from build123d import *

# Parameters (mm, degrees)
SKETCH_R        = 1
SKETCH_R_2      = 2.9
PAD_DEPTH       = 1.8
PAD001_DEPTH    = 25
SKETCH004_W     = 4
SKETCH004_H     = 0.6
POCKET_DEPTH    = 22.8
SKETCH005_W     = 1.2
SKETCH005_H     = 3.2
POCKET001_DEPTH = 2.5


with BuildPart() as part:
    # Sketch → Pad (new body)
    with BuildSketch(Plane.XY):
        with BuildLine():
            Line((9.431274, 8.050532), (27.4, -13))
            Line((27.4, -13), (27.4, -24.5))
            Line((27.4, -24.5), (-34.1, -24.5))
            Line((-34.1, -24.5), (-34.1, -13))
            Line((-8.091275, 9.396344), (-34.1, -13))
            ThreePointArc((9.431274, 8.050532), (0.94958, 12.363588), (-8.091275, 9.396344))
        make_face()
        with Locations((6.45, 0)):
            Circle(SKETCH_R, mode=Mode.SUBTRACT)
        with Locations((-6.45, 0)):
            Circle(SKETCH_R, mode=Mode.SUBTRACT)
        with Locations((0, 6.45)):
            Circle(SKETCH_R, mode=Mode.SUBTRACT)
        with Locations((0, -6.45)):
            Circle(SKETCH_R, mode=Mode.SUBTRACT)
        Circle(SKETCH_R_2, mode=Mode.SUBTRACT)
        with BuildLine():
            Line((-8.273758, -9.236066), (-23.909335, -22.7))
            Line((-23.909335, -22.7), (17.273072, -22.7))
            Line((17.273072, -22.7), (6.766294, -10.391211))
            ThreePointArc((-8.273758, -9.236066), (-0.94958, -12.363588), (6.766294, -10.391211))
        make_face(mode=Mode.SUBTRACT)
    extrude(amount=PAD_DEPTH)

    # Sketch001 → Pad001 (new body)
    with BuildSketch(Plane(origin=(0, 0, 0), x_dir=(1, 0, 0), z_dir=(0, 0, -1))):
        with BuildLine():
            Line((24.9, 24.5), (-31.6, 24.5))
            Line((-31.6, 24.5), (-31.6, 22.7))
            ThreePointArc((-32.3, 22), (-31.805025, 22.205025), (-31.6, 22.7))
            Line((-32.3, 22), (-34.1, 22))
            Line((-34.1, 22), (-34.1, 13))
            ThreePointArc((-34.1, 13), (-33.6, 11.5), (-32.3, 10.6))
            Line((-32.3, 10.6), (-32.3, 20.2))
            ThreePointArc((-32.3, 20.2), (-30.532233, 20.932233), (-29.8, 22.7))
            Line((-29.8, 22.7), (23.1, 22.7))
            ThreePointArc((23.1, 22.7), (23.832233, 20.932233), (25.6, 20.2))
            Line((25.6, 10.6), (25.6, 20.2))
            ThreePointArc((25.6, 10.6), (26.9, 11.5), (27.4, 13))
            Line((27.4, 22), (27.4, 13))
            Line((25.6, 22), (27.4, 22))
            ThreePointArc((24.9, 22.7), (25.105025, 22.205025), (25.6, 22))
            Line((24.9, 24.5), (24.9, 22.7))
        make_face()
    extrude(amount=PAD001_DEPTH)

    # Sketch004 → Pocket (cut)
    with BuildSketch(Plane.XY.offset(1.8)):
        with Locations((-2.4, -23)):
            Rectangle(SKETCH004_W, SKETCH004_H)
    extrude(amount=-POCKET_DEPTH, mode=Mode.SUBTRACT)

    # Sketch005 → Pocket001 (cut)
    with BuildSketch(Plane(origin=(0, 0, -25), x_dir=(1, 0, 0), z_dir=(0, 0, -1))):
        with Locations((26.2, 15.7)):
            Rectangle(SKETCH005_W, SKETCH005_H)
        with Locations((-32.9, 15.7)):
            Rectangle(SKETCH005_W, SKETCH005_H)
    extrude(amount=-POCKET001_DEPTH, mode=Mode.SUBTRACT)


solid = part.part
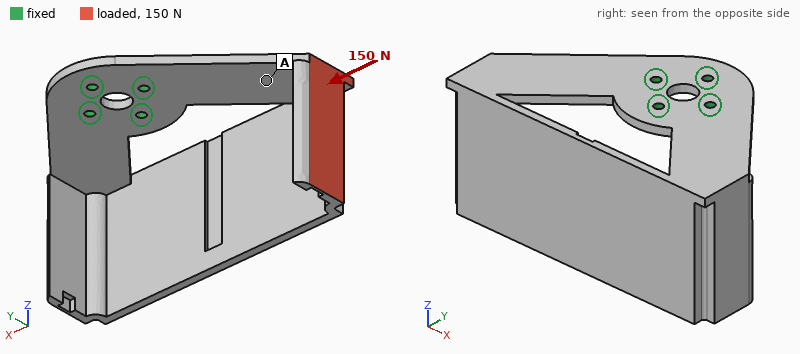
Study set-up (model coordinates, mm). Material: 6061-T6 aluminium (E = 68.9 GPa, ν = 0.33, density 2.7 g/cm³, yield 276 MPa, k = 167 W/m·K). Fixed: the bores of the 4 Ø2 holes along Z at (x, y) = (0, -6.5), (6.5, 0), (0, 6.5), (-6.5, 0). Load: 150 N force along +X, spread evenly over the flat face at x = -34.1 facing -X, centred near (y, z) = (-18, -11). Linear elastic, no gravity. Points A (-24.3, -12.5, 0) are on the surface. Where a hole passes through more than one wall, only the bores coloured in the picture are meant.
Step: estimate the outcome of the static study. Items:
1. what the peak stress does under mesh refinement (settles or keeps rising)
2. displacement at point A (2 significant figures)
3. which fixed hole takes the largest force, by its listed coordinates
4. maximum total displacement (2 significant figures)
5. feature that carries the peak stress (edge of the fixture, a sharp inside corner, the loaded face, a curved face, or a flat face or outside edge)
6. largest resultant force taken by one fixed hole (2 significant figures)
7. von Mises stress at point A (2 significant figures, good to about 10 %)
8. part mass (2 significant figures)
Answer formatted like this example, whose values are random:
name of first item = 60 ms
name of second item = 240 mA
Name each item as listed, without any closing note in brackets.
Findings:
what the peak stress does under mesh refinement = keeps rising
displacement at point A = 0.27 mm
which fixed hole takes the largest force, by its listed coordinates = (0, -6.5)
maximum total displacement = 0.72 mm
feature that carries the peak stress = edge of the fixture
largest resultant force taken by one fixed hole = 220 N
von Mises stress at point A = 19 MPa
part mass = 16 g
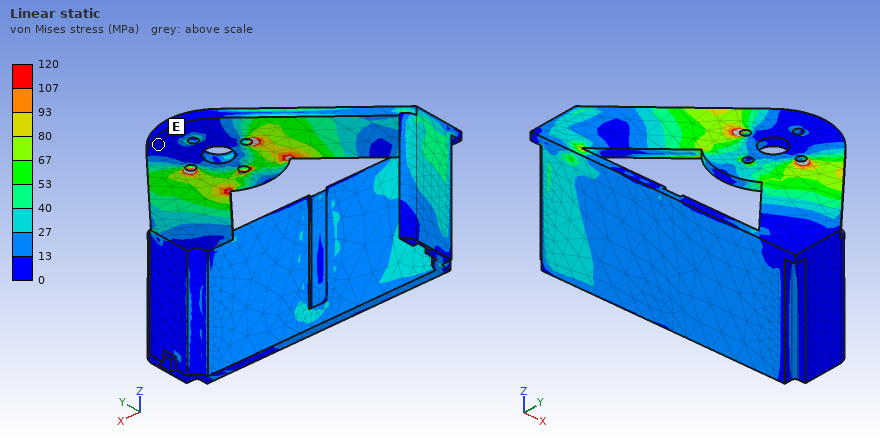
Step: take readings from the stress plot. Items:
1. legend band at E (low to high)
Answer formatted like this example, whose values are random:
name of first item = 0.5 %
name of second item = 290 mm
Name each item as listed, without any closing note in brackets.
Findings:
legend band at E = 0 to 13 MPa
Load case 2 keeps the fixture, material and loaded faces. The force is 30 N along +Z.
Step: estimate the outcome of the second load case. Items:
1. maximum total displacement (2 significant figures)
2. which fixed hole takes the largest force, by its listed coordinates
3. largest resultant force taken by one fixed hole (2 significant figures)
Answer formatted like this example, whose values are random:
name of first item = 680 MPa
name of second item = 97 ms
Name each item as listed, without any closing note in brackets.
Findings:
maximum total displacement = 0.45 mm
which fixed hole takes the largest force, by its listed coordinates = (-6.5, 0)
largest resultant force taken by one fixed hole = 53 N
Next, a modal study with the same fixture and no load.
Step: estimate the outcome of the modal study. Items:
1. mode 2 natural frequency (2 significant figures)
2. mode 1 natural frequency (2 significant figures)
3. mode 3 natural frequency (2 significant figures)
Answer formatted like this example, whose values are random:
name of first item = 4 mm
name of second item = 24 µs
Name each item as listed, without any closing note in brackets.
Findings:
mode 2 natural frequency = 660 Hz
mode 1 natural frequency = 540 Hz
mode 3 natural frequency = 1400 Hz
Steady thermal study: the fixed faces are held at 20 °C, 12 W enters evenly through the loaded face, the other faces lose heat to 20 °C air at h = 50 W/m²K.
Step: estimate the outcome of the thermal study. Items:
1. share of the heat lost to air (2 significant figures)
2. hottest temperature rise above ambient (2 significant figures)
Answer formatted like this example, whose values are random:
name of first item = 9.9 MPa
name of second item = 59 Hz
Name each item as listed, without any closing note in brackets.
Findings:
share of the heat lost to air = 51 %
hottest temperature rise above ambient = 46 K
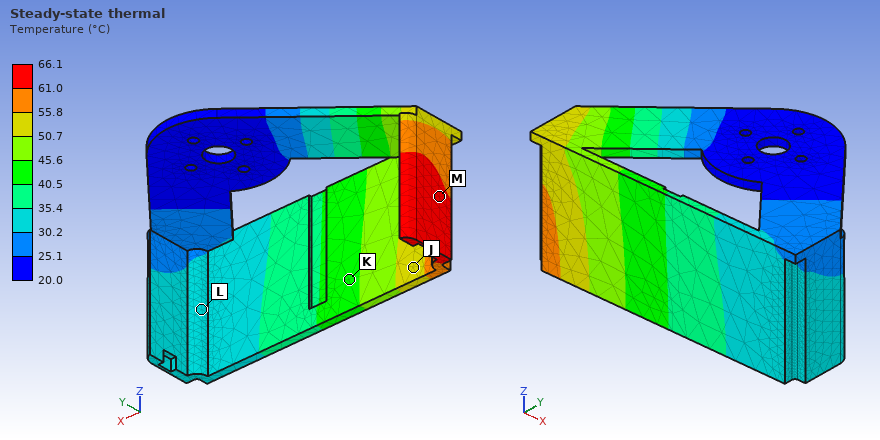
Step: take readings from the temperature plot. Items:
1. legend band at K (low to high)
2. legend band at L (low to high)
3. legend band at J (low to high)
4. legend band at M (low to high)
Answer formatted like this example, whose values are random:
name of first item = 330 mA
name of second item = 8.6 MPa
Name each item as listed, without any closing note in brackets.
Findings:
legend band at K = 40.5 to 45.6 °C
legend band at L = 30.2 to 35.4 °C
legend band at J = 50.7 to 55.8 °C
legend band at M = 61.0 to 66.1 °C
